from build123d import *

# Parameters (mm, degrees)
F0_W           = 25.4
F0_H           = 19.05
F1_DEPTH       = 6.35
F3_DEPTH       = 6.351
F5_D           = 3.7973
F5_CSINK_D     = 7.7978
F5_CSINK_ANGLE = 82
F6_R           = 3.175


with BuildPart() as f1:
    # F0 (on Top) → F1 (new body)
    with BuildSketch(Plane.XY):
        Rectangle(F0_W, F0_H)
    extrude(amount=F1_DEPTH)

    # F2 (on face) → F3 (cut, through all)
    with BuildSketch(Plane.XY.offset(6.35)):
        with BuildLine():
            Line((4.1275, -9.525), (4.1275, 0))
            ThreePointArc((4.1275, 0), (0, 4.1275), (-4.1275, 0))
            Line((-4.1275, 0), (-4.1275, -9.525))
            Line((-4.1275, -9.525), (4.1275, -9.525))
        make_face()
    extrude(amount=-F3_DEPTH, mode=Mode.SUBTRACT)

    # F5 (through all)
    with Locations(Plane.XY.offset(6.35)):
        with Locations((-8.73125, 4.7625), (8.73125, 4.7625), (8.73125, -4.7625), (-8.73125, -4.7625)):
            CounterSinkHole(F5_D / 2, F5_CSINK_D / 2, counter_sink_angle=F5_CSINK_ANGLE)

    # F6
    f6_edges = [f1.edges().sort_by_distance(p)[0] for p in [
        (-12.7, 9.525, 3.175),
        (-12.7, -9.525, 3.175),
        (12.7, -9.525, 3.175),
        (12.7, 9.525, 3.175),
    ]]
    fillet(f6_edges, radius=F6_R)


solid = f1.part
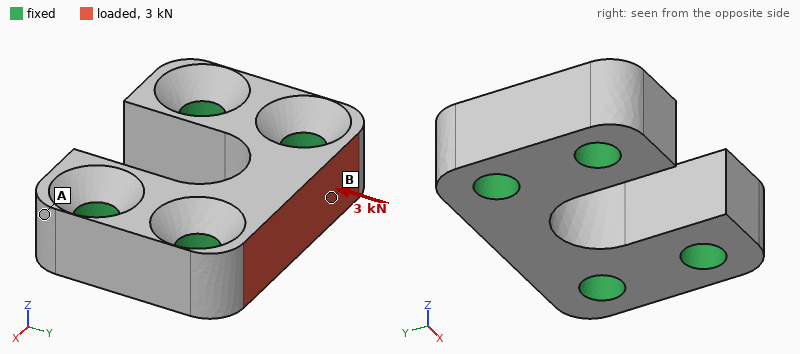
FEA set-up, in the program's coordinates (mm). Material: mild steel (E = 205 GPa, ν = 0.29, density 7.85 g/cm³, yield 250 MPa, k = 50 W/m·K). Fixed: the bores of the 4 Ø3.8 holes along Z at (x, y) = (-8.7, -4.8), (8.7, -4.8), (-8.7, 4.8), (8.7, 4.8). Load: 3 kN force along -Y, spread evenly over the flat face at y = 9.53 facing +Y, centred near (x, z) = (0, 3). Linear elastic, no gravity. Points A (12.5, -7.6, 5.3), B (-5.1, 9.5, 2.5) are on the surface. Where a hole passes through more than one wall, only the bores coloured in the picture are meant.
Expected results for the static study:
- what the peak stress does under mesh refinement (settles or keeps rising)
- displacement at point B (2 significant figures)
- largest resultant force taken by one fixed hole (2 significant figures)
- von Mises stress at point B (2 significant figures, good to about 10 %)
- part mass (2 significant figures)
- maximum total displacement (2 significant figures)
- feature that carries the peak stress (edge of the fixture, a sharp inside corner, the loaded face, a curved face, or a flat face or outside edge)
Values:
keeps rising
1.5 µm
1.2 kN
29 MPa
15 g
2.7 µm
edge of the fixture
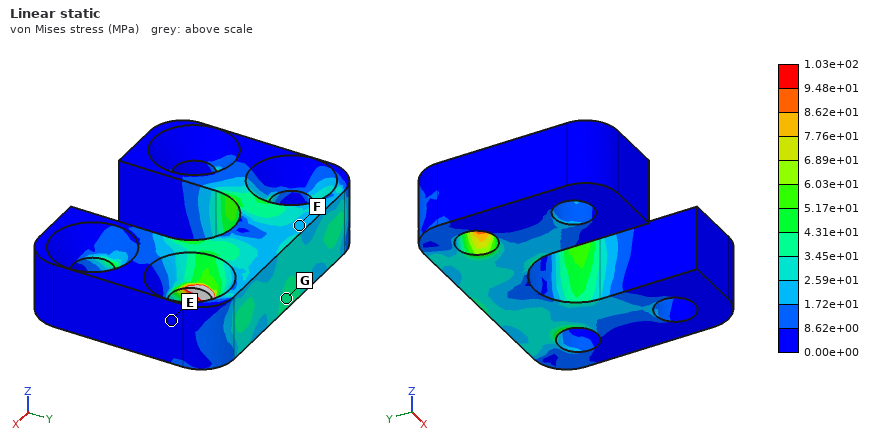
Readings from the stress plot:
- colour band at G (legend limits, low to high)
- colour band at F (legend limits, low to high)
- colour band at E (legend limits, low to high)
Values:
3.45e+01 to 4.31e+01 MPa
1.72e+01 to 2.59e+01 MPa
0.00e+00 to 8.62e+00 MPa
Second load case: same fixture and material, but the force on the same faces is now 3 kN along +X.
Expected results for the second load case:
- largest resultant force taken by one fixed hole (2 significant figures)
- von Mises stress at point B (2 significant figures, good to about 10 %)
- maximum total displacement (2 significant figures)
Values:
1.6 kN
46 MPa
1.8 µm
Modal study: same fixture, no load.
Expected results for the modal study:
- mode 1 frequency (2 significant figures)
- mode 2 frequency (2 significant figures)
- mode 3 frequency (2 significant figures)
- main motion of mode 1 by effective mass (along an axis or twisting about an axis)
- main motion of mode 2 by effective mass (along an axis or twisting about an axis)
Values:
66 kHz
93 kHz
100 kHz
along Z
along Y
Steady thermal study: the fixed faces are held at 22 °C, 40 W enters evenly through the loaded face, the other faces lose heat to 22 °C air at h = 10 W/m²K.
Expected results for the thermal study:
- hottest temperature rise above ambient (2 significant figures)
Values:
51 K
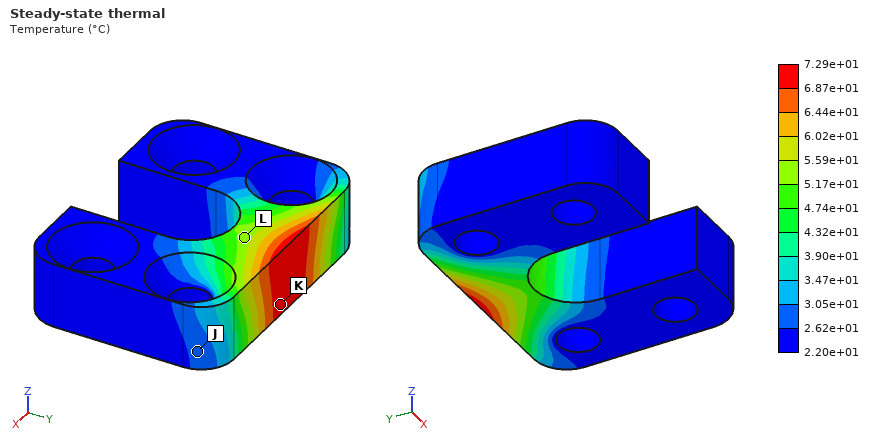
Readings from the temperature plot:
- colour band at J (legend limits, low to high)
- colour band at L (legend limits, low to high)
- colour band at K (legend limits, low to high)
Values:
2.62e+01 to 3.05e+01 °C
5.17e+01 to 5.59e+01 °C
6.87e+01 to 7.29e+01 °C
